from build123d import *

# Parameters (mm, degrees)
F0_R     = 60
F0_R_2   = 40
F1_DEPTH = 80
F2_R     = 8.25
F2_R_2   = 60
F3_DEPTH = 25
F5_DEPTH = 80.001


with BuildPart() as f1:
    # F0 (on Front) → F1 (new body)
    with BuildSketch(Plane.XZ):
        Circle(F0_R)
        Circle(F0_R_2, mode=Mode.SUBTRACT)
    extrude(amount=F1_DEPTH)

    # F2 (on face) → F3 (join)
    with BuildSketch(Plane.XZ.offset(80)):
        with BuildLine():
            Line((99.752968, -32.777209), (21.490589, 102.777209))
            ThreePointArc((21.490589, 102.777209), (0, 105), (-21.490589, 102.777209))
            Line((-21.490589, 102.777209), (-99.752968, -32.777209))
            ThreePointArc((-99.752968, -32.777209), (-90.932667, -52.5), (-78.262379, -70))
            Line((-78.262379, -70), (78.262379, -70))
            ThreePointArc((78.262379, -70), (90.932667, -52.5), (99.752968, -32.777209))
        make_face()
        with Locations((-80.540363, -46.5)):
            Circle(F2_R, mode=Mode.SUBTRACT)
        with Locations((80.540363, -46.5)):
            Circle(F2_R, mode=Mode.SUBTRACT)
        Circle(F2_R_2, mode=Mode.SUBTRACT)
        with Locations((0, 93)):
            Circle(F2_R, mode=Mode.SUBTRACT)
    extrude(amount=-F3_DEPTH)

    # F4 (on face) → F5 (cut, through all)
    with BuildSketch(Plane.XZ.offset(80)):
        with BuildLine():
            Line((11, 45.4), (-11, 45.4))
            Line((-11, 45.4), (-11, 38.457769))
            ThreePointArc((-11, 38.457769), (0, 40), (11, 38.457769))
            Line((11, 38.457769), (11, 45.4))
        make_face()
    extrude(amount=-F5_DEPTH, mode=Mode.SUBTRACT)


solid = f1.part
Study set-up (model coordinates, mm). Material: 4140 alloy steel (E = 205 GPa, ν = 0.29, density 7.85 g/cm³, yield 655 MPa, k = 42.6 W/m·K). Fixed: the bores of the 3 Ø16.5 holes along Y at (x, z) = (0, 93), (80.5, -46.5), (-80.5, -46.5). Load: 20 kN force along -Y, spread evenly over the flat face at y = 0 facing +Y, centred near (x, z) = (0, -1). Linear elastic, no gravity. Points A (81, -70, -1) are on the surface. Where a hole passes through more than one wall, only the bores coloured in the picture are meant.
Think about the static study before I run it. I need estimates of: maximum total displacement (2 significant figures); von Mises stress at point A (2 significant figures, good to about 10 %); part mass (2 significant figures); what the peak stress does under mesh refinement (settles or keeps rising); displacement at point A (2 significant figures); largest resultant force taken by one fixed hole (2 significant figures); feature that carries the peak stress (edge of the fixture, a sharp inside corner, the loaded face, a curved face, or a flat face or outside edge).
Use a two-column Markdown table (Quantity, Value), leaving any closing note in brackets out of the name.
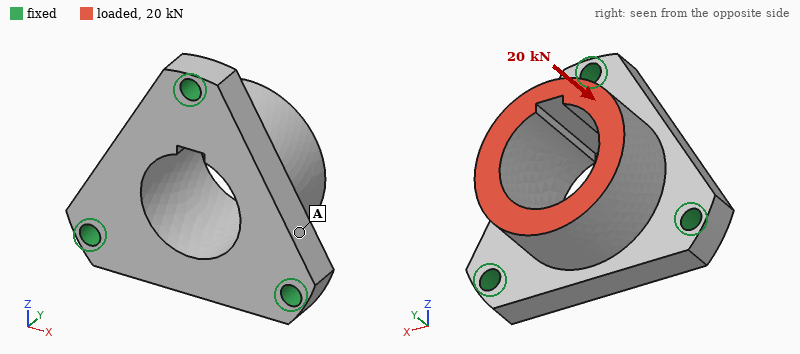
| Quantity | Value |
|---|---|
| maximum total displacement | 7.7 µm |
| von Mises stress at point A | 5.4 MPa |
| part mass | 6.1 kg |
| what the peak stress does under mesh refinement | keeps rising |
| displacement at point A | 3.9 µm |
| largest resultant force taken by one fixed hole | 7.1 kN |
| feature that carries the peak stress | edge of the fixture |
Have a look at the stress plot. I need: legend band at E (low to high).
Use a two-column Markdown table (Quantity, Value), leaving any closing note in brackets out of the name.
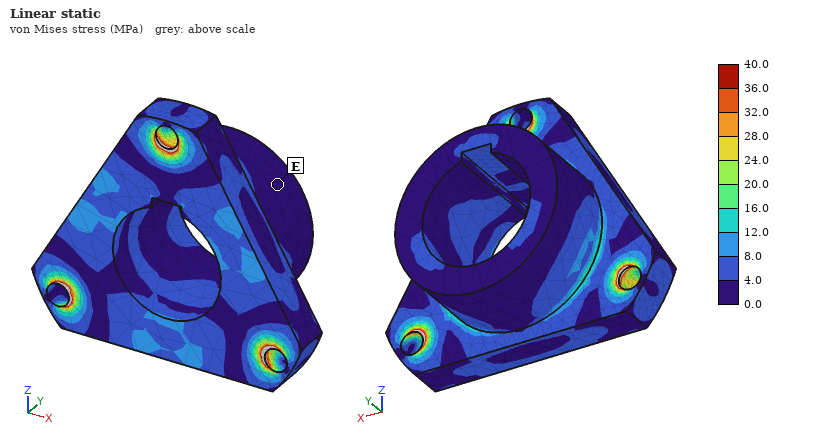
| Quantity | Value |
|---|---|
| legend band at E | 0.0 to 4.0 MPa |
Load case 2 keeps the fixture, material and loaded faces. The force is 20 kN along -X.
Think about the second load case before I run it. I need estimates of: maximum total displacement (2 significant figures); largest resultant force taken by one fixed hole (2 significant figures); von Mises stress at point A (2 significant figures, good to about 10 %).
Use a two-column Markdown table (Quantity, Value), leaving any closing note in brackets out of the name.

| Quantity | Value |
|---|---|
| maximum total displacement | 25 µm |
| largest resultant force taken by one fixed hole | 12 kN |
| von Mises stress at point A | 13 MPa |
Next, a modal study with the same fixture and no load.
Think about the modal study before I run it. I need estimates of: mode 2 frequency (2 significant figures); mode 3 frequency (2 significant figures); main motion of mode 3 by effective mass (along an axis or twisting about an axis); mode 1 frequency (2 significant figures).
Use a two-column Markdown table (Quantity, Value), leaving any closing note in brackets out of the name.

| Quantity | Value |
|---|---|
| mode 2 frequency | 3800 Hz |
| mode 3 frequency | 4000 Hz |
| main motion of mode 3 by effective mass | along Y |
| mode 1 frequency | 3700 Hz |
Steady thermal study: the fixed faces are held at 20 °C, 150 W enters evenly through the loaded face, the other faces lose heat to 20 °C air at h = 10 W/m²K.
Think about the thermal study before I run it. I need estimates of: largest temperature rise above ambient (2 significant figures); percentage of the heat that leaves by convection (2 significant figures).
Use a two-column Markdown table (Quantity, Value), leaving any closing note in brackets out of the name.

| Quantity | Value |
|---|---|
| largest temperature rise above ambient | 59 K |
| percentage of the heat that leaves by convection | 16 % |
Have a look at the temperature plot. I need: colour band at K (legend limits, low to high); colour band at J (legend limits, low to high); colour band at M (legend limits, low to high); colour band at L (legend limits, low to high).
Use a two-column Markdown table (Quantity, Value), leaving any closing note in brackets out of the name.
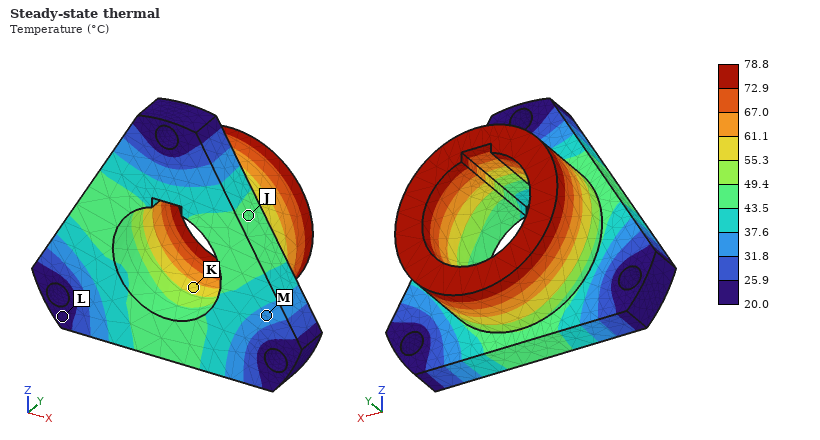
| Quantity | Value |
|---|---|
| colour band at K | 55.3 to 61.1 °C |
| colour band at J | 43.5 to 49.4 °C |
| colour band at M | 31.8 to 37.6 °C |
| colour band at L | 20.0 to 25.9 °C |
